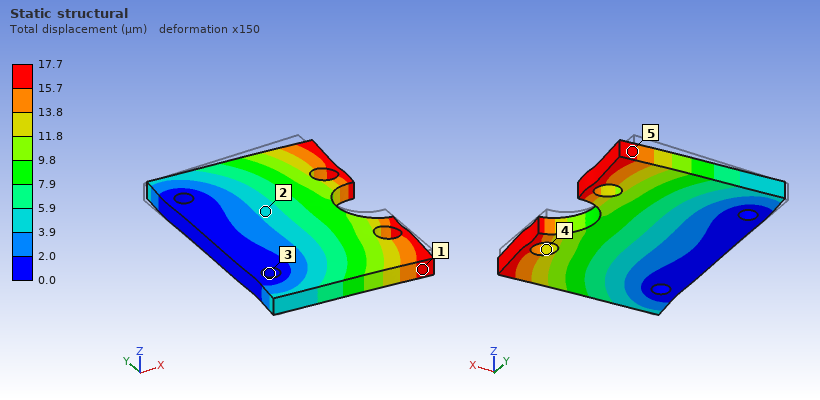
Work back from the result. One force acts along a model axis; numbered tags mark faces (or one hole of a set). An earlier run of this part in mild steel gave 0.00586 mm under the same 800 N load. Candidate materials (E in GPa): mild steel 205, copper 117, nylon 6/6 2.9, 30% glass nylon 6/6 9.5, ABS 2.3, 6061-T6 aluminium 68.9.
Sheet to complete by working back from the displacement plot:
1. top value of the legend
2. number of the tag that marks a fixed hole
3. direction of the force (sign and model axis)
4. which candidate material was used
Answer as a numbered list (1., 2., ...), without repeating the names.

1. 17.7 µm
2. 3
3. -Y
4. 6061-T6 aluminium
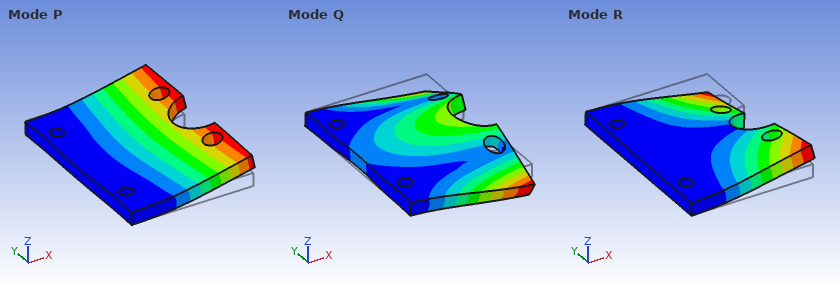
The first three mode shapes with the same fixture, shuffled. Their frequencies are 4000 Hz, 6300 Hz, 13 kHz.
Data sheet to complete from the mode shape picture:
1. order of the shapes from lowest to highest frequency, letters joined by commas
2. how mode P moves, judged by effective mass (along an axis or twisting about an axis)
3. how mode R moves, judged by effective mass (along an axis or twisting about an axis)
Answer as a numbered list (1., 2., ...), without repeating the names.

1. P, R, Q
2. along Z
3. twisting about X
